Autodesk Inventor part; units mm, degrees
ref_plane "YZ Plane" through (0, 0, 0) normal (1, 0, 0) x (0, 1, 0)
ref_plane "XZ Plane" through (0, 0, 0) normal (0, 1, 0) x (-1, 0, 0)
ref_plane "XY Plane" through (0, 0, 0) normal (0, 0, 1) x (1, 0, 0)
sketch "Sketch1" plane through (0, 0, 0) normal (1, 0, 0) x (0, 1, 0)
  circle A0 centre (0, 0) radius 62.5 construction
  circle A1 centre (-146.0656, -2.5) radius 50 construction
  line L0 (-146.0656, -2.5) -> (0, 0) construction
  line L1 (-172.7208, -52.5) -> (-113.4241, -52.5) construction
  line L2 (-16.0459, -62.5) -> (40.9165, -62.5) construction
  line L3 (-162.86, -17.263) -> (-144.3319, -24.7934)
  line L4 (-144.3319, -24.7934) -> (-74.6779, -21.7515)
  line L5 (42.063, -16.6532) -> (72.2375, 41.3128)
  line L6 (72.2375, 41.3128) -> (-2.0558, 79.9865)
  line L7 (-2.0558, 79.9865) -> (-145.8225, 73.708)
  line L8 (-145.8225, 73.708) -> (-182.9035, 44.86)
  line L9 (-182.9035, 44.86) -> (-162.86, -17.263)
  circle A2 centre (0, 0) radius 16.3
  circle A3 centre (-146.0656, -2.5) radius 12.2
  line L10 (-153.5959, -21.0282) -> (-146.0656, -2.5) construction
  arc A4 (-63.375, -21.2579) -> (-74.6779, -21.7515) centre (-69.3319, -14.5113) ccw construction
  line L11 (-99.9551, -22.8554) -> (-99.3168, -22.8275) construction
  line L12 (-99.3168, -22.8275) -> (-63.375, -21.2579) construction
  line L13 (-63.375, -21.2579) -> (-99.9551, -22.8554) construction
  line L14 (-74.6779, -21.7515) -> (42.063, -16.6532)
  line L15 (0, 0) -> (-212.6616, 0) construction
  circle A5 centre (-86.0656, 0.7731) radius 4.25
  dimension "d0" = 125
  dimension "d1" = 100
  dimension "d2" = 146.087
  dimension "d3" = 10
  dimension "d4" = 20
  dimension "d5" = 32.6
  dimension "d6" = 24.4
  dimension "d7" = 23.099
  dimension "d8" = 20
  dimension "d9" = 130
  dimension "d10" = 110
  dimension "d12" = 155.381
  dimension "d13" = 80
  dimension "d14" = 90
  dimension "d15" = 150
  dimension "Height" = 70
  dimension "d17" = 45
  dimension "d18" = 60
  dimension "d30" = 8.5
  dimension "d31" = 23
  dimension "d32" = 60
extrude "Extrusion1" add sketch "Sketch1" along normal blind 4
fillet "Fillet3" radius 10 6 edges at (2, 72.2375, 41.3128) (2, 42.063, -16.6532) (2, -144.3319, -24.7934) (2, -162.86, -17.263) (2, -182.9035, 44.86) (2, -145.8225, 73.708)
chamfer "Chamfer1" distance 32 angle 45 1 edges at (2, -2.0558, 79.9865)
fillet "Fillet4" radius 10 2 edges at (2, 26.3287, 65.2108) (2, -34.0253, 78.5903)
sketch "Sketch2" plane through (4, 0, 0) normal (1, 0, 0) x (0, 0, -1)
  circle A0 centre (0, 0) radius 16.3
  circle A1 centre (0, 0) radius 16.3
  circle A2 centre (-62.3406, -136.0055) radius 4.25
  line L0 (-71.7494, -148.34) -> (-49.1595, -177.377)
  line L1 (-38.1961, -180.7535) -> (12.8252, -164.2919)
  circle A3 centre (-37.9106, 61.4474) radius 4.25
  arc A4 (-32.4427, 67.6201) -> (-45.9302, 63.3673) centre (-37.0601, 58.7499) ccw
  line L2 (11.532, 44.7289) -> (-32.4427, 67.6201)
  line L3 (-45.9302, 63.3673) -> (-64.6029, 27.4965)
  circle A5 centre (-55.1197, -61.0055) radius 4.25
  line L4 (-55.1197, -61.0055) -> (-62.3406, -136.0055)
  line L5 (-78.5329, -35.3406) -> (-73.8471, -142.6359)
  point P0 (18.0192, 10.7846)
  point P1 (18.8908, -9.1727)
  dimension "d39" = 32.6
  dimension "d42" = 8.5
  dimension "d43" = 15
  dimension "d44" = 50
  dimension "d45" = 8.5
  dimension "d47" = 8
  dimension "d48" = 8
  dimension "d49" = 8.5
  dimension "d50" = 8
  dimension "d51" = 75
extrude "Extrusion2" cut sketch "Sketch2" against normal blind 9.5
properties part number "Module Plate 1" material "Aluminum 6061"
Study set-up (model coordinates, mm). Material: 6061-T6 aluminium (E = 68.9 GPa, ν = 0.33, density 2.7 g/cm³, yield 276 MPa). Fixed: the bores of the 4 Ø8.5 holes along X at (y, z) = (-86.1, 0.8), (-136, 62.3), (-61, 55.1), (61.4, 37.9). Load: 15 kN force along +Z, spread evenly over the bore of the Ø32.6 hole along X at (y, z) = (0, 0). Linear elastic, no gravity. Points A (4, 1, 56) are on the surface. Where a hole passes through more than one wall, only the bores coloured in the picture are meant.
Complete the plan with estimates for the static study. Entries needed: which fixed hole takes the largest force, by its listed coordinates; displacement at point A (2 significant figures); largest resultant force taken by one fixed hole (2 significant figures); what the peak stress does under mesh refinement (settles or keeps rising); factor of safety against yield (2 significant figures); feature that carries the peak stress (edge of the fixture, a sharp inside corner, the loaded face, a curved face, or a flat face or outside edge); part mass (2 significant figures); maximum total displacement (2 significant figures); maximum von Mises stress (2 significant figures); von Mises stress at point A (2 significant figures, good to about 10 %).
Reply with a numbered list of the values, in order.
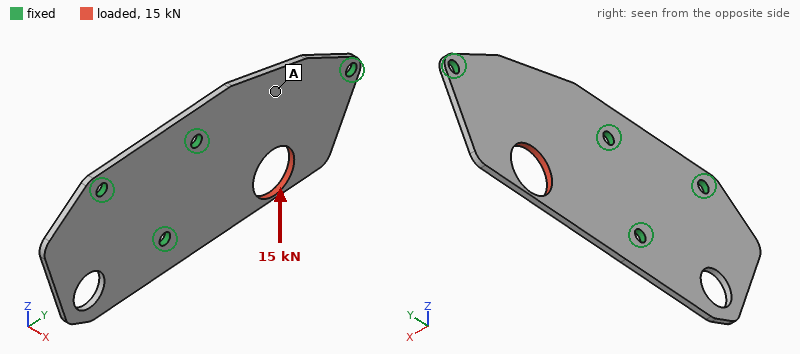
1. (-61, 55.1)
2. 0.074 mm
3. 8.4 kN
4. settles
5. 0.48
6. a flat face or outside edge
7. 210 g
8. 0.23 mm
9. 580 MPa
10. 28 MPa
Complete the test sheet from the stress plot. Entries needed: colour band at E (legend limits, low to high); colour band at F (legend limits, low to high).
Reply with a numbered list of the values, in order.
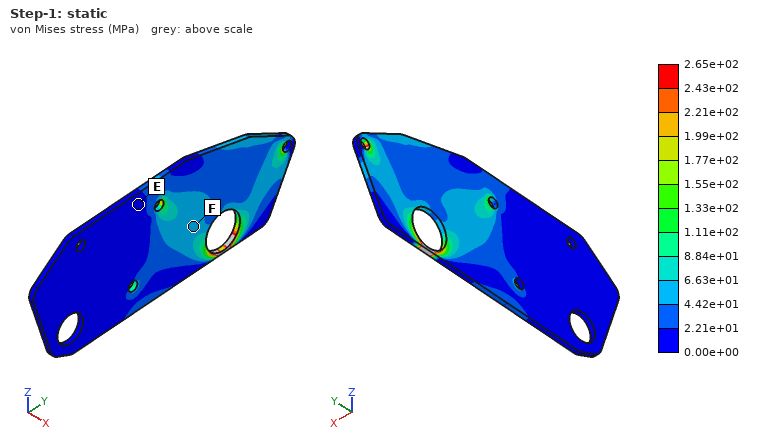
1. 0.00e+00 to 2.21e+01 MPa
2. 4.42e+01 to 6.63e+01 MPa
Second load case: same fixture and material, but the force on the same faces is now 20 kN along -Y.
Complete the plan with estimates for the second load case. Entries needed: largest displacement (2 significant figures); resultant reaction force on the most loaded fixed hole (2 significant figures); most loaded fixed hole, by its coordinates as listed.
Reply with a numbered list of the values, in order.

1. 0.15 mm
2. 8.3 kN
3. (61.4, 37.9)
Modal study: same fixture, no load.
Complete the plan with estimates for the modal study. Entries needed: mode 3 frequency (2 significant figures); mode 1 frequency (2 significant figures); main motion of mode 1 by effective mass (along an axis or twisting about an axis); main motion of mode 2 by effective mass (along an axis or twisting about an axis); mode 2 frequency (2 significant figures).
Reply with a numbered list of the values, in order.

1. 1400 Hz
2. 910 Hz
3. along X
4. along X
5. 970 Hz
